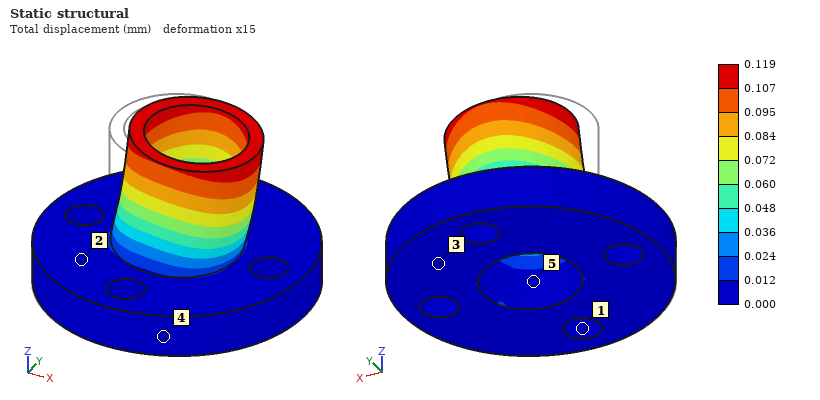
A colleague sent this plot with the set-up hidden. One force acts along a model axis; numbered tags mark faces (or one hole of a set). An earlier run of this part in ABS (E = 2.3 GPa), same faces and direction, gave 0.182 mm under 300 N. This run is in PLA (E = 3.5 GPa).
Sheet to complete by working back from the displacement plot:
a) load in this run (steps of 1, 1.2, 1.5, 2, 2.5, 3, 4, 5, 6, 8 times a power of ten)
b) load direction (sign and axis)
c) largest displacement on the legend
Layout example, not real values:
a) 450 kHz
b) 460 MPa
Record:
a) 300 N
b) +X
c) 0.119 mm
